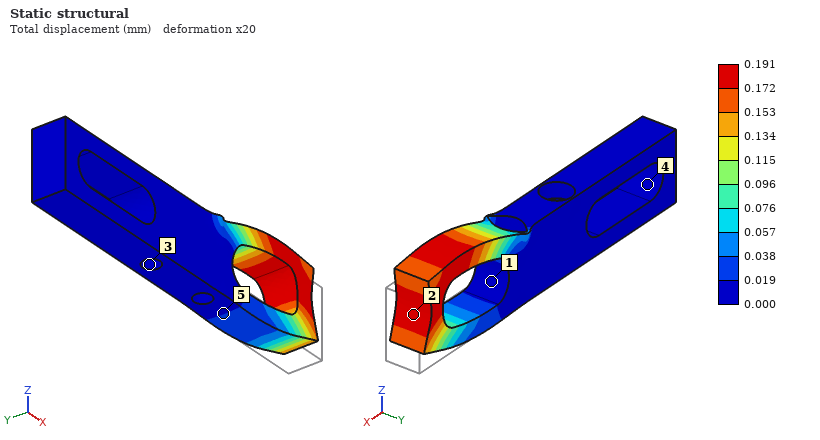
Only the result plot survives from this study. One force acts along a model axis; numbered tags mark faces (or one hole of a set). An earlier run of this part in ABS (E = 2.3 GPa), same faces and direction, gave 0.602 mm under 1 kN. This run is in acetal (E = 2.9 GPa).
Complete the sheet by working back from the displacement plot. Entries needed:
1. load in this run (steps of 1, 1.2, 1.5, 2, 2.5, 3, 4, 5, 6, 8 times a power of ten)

400 N
